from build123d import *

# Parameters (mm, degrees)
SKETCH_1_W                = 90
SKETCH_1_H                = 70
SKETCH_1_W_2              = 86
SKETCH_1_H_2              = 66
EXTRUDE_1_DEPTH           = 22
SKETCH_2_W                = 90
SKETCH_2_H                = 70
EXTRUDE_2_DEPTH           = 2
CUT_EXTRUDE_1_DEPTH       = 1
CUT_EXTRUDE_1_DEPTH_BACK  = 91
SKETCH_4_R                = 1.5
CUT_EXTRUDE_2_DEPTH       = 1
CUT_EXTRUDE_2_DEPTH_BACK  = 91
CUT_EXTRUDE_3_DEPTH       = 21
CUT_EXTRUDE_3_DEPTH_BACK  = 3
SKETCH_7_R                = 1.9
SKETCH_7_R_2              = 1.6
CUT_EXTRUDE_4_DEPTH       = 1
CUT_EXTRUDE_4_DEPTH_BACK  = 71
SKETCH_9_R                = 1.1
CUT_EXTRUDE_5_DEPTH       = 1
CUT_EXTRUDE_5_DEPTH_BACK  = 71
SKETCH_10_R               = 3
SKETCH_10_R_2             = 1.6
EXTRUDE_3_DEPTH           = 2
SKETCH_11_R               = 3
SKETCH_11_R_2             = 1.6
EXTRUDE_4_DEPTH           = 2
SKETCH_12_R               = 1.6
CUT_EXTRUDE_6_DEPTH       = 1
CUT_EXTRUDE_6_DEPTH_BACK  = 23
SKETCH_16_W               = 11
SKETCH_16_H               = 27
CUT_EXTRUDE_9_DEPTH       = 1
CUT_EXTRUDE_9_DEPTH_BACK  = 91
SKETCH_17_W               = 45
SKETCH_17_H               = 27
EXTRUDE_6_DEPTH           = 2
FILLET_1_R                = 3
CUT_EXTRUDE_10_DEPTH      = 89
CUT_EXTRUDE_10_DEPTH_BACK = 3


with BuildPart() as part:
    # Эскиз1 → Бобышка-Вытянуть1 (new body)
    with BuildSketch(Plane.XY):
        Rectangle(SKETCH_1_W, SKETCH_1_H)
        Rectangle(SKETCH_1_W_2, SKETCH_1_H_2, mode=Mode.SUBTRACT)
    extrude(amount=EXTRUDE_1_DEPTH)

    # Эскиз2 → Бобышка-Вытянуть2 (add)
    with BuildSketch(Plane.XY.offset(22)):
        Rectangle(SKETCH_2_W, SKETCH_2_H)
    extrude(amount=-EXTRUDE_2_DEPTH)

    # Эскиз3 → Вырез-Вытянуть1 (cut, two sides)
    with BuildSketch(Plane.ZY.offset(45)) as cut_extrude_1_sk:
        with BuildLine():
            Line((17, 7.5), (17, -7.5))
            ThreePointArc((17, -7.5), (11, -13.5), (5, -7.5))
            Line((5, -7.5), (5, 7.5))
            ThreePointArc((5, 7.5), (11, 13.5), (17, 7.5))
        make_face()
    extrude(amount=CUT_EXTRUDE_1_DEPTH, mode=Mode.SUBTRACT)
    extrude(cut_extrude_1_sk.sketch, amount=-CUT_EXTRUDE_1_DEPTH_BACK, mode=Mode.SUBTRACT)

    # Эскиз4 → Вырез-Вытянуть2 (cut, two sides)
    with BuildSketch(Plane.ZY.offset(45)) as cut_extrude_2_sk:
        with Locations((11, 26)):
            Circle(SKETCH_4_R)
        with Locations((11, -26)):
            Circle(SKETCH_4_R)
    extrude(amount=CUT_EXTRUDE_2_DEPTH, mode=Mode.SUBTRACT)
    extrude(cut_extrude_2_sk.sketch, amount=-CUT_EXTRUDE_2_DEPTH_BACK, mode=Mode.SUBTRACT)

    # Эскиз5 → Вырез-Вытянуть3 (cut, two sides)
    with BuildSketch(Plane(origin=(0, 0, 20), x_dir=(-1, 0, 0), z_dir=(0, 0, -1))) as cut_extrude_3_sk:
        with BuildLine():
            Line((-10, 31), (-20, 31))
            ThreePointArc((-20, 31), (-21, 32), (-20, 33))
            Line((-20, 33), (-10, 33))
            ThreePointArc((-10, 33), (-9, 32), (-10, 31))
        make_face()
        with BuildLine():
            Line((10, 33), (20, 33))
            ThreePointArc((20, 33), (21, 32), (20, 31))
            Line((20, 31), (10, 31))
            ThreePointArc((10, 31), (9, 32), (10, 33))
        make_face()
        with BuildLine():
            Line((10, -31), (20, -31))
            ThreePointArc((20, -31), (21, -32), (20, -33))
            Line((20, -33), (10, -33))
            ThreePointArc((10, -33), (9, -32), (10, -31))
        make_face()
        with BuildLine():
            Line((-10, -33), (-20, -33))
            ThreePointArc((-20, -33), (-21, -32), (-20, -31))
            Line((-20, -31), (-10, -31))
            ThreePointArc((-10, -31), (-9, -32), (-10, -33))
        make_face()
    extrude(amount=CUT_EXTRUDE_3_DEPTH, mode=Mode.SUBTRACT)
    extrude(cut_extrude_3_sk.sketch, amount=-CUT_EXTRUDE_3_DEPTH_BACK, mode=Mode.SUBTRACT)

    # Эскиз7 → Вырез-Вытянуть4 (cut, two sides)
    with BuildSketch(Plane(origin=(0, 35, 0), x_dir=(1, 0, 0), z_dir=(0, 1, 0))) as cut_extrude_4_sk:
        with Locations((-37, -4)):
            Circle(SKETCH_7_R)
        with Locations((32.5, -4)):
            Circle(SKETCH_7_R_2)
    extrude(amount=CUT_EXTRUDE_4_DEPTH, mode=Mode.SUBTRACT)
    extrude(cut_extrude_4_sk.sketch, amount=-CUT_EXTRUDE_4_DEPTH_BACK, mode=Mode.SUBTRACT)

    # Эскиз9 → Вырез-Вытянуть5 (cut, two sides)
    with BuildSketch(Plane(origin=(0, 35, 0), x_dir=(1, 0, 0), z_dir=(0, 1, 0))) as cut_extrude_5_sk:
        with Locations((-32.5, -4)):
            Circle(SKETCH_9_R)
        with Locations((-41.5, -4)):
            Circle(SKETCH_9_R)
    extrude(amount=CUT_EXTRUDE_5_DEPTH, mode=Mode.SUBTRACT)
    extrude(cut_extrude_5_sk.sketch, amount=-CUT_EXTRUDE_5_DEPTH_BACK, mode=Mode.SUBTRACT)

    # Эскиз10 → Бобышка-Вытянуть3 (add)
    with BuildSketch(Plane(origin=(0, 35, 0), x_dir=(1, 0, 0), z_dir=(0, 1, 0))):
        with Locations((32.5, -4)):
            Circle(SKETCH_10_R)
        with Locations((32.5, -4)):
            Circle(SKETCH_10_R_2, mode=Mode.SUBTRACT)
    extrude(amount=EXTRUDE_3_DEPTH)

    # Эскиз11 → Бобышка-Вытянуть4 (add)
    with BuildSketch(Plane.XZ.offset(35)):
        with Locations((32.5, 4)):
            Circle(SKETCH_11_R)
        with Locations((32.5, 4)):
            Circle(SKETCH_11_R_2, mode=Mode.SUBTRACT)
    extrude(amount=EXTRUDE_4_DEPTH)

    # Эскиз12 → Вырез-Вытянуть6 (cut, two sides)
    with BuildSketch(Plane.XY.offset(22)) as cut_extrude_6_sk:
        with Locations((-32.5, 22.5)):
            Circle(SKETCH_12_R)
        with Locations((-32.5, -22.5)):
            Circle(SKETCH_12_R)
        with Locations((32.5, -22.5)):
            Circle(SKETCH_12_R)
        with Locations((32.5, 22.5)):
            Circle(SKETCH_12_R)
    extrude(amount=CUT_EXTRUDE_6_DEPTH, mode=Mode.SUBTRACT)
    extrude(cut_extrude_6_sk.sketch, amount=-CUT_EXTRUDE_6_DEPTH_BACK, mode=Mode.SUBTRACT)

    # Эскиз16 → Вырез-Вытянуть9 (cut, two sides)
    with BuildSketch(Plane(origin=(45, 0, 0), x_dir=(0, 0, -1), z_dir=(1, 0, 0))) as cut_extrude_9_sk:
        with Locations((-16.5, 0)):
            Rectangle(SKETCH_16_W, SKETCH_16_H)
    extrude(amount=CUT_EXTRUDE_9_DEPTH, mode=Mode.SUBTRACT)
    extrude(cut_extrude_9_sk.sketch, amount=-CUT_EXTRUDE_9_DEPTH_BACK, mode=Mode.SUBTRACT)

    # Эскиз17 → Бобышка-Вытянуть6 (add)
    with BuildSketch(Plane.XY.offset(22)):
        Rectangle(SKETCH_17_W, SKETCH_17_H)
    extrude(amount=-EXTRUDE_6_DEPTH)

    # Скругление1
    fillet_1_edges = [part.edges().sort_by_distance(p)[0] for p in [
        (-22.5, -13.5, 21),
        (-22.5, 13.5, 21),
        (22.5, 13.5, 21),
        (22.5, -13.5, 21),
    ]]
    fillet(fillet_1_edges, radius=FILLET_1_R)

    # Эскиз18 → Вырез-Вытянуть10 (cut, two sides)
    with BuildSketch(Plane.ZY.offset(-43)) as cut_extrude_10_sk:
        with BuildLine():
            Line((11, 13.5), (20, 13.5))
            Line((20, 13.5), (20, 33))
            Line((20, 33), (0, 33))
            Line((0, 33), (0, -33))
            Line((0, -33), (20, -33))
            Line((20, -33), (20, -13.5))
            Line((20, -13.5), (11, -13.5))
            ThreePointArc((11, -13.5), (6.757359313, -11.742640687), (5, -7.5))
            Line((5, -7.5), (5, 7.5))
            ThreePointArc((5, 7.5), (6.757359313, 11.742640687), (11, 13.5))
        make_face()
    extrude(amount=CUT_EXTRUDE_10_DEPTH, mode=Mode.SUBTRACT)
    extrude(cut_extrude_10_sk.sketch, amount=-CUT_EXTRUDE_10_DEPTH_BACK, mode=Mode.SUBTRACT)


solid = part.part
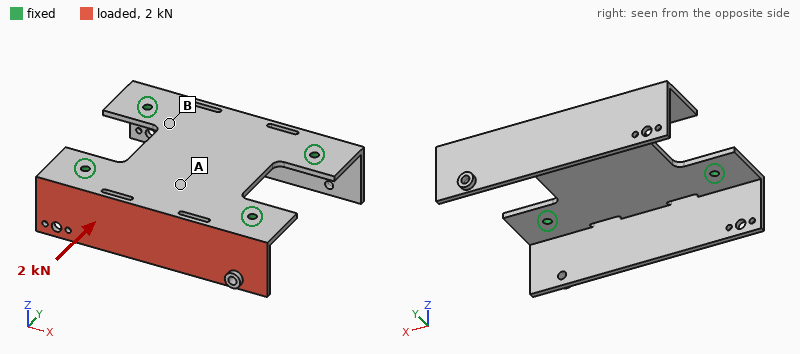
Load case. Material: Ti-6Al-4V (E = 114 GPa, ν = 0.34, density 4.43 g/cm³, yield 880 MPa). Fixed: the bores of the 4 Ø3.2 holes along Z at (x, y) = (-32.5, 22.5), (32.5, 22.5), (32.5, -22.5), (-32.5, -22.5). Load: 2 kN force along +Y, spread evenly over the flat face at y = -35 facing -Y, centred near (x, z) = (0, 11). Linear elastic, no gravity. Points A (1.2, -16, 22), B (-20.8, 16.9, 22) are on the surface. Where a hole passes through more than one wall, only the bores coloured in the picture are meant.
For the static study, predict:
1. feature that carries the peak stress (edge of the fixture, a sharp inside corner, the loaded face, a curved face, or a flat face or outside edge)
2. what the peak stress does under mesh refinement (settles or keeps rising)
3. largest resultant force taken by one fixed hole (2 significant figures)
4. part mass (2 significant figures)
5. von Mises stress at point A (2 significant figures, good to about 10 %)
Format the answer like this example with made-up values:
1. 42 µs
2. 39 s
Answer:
1. edge of the fixture
2. keeps rising
3. 760 N
4. 76 g
5. 120 MPa
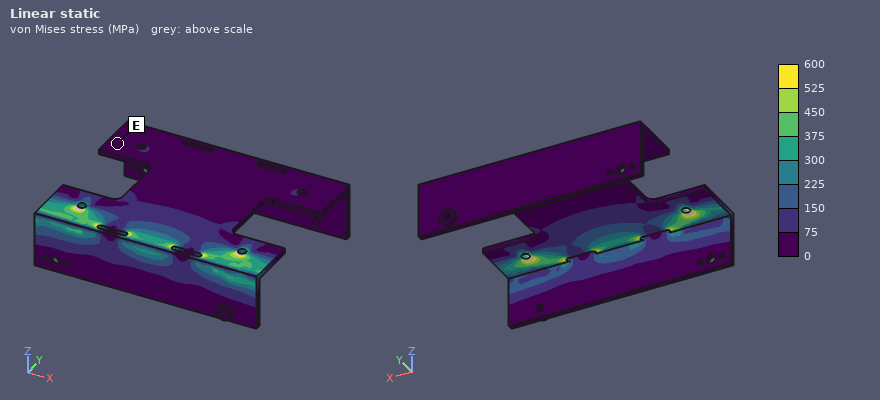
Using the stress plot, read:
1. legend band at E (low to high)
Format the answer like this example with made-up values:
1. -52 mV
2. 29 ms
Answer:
1. 0 to 75 MPa
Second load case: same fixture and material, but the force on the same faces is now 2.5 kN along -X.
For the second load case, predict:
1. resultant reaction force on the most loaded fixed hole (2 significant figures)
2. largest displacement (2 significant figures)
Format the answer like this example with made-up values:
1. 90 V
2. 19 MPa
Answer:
1. 1.3 kN
2. 0.19 mm
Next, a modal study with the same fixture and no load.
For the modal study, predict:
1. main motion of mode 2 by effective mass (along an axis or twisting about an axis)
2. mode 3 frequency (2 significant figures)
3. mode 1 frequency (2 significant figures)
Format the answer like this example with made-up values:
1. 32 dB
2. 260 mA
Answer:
1. along Y
2. 2500 Hz
3. 1700 Hz
